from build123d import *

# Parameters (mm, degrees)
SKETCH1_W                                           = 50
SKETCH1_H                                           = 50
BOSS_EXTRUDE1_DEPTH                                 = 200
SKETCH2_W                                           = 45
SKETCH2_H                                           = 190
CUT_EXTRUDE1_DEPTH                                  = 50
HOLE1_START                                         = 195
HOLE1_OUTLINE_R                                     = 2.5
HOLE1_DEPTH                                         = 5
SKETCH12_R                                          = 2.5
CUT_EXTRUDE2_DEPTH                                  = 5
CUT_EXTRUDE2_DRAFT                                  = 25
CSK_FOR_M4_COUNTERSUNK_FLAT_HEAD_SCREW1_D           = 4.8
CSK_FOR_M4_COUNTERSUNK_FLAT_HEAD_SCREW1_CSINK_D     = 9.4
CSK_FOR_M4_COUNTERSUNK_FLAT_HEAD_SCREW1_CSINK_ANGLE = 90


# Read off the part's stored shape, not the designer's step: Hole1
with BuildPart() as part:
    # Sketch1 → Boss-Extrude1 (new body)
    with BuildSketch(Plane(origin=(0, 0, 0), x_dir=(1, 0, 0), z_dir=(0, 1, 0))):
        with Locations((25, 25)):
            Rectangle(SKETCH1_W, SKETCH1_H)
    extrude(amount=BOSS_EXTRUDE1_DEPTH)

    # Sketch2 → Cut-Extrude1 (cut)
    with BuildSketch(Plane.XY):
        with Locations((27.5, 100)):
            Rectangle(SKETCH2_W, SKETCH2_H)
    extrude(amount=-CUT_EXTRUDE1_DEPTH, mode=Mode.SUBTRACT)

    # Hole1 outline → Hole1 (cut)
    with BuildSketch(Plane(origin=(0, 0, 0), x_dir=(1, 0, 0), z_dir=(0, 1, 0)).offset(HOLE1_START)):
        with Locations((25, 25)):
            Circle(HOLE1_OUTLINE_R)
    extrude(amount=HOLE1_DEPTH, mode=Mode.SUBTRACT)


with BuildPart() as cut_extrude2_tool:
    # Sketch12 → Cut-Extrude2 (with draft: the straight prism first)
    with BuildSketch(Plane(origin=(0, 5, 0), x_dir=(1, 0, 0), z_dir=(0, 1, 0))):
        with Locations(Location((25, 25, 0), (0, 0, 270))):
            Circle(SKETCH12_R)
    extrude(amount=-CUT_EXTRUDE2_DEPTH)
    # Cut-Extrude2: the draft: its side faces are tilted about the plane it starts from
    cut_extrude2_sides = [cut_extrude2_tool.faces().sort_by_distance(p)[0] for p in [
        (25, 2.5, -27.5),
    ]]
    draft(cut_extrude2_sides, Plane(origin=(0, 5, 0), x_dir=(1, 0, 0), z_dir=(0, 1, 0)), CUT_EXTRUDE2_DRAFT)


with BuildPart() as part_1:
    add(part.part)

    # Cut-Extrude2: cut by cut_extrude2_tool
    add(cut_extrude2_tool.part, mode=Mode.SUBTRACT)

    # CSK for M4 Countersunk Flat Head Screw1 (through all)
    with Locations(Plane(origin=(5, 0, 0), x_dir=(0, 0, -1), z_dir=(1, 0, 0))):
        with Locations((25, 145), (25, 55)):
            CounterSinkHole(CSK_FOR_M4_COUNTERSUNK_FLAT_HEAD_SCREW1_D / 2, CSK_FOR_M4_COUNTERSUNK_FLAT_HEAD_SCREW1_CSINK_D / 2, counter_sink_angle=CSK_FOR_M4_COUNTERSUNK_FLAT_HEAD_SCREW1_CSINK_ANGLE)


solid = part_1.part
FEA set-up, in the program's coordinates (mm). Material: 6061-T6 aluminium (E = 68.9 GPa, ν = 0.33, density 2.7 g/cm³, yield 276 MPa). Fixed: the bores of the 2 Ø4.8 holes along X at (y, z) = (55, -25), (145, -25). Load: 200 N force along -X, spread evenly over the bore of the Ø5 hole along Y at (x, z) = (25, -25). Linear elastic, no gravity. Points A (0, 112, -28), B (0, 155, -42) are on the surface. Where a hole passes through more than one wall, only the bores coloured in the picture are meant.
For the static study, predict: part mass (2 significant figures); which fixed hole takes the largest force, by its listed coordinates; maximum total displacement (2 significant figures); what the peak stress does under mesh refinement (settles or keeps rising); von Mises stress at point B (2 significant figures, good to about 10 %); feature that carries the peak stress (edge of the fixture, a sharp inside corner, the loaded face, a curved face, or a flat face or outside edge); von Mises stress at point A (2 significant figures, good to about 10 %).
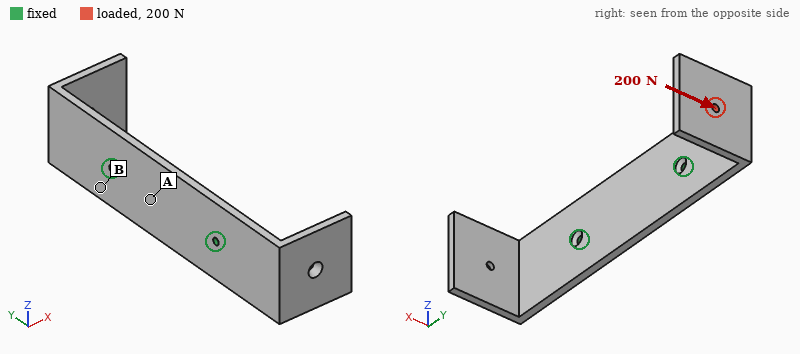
190 g
(145, -25)
0.62 mm
keeps rising
36 MPa
edge of the fixture
7.5 MPa
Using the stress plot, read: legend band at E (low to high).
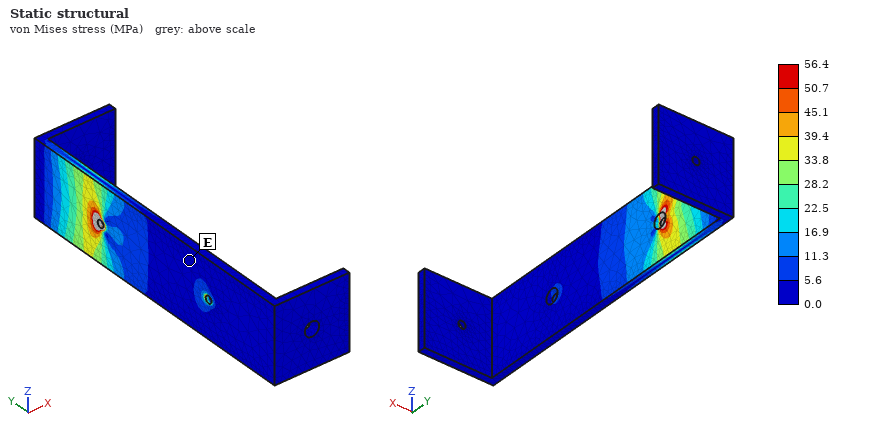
0.0 to 5.6 MPa
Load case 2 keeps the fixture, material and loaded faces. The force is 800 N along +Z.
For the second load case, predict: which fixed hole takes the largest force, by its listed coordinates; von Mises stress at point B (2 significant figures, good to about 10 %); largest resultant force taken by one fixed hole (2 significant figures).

(145, -25)
55 MPa
1.2 kN
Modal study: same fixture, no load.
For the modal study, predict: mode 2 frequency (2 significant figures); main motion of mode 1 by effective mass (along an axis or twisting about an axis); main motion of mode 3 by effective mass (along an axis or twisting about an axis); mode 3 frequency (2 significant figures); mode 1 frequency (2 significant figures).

480 Hz
along X
along Z
760 Hz
460 Hz
